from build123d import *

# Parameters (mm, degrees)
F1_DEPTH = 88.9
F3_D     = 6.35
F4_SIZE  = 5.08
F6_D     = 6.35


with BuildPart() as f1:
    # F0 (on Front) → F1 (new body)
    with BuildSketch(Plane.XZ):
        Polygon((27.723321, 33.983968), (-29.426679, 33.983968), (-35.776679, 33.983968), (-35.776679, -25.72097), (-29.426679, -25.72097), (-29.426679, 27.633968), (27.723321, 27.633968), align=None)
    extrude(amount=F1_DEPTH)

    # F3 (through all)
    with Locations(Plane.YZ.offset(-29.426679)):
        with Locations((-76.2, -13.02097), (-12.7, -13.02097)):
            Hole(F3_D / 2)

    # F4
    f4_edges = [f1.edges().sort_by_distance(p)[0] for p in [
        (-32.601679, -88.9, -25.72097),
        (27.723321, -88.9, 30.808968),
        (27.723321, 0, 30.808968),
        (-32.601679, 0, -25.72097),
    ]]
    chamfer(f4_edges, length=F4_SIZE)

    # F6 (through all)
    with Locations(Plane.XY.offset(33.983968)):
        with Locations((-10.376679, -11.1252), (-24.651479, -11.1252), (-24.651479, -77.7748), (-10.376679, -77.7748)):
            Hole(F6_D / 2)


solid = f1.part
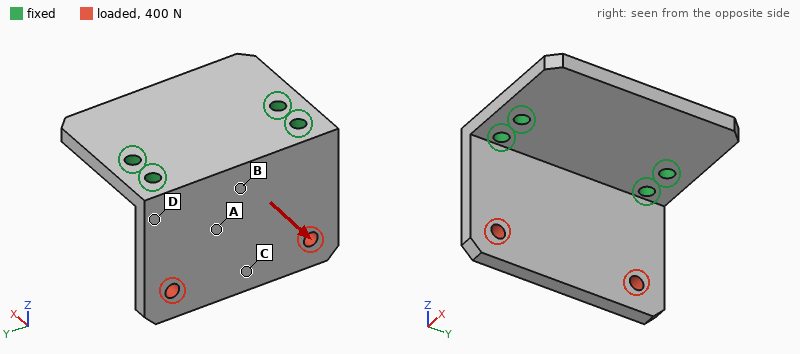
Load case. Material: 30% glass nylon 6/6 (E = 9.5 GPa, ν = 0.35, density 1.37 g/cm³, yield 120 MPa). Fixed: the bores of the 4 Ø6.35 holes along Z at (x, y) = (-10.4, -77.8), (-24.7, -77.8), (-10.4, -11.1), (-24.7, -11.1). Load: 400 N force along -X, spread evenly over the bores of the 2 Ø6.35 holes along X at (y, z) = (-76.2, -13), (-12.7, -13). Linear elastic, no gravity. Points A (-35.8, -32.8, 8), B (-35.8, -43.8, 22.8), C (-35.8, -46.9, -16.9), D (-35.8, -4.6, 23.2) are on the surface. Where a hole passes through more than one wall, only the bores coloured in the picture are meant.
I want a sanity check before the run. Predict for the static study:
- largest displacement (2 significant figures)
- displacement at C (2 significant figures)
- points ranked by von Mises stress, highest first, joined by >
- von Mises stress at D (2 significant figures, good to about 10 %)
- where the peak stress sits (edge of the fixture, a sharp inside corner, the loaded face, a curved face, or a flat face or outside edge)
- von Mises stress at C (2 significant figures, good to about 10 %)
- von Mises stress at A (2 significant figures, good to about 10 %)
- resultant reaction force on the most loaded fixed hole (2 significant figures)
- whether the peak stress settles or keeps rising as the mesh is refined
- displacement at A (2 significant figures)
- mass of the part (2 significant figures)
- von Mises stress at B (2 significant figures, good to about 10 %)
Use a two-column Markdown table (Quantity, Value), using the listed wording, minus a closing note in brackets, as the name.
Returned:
| Quantity | Value |
|---|---|
| largest displacement | 1.2 mm |
| displacement at C | 0.95 mm |
| points ranked by von Mises stress, highest first, joined by > | D > B > A > C |
| von Mises stress at D | 26 MPa |
| where the peak stress sits | edge of the fixture |
| von Mises stress at C | 4.4 MPa |
| von Mises stress at A | 12 MPa |
| resultant reaction force on the most loaded fixed hole | 280 N |
| whether the peak stress settles or keeps rising as the mesh is refined | keeps rising |
| displacement at A | 0.36 mm |
| mass of the part | 88 g |
| von Mises stress at B | 19 MPa |
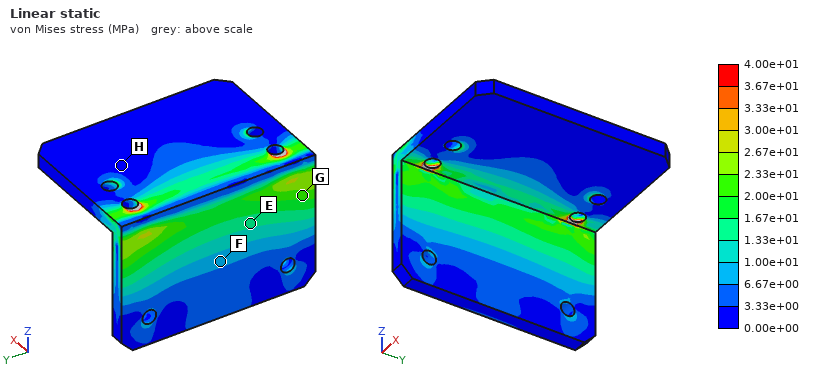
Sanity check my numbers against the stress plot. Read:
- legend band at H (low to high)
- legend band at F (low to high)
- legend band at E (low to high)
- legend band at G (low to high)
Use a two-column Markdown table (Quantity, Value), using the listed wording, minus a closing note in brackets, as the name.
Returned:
| Quantity | Value |
|---|---|
| legend band at H | 0.00e+00 to 3.33e+00 MPa |
| legend band at F | 6.67e+00 to 1.00e+01 MPa |
| legend band at E | 1.33e+01 to 1.67e+01 MPa |
| legend band at G | 2.00e+01 to 2.33e+01 MPa |
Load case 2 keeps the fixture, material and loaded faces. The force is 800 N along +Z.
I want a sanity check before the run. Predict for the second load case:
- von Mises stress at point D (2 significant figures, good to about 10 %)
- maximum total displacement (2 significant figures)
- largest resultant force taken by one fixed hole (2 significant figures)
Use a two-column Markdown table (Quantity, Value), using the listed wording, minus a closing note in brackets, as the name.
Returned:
| Quantity | Value |
|---|---|
| von Mises stress at point D | 2.3 MPa |
| maximum total displacement | 0.11 mm |
| largest resultant force taken by one fixed hole | 440 N |
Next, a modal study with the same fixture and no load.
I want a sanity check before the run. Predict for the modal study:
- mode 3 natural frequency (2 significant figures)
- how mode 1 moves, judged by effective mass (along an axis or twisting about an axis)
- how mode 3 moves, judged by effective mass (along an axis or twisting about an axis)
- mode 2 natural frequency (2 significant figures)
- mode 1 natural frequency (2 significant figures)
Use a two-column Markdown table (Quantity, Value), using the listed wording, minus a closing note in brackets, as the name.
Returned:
| Quantity | Value |
|---|---|
| mode 3 natural frequency | 1600 Hz |
| how mode 1 moves, judged by effective mass | along X |
| how mode 3 moves, judged by effective mass | along Z |
| mode 2 natural frequency | 1400 Hz |
| mode 1 natural frequency | 720 Hz |
